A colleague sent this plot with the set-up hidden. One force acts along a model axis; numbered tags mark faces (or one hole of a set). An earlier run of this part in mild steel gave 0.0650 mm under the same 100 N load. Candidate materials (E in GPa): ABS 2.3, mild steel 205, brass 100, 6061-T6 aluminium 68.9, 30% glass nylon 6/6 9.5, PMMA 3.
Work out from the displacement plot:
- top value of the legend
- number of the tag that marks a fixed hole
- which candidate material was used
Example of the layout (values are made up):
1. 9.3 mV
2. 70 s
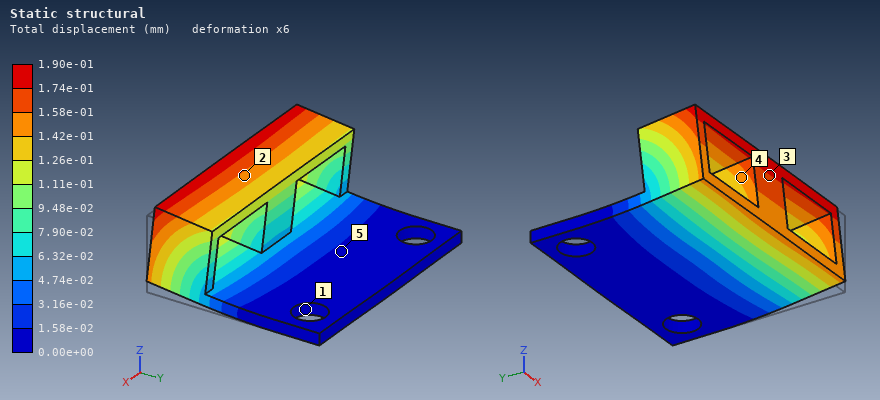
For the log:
1. 1.90e-01 mm
2. 1
3. 6061-T6 aluminium
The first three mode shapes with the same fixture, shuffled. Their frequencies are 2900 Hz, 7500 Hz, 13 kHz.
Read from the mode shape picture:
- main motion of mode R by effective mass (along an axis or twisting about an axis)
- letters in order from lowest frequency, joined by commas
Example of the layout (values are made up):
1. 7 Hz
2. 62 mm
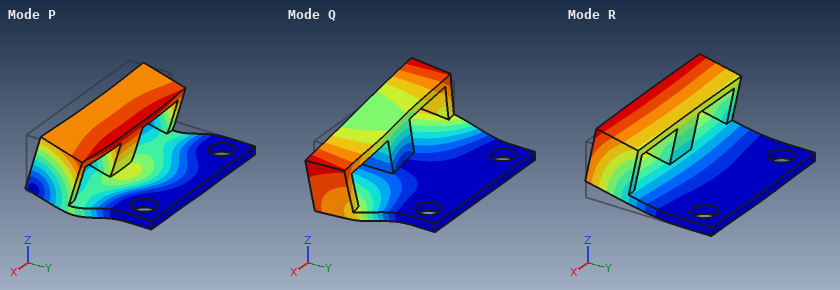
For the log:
1. along Z
2. R, Q, P
